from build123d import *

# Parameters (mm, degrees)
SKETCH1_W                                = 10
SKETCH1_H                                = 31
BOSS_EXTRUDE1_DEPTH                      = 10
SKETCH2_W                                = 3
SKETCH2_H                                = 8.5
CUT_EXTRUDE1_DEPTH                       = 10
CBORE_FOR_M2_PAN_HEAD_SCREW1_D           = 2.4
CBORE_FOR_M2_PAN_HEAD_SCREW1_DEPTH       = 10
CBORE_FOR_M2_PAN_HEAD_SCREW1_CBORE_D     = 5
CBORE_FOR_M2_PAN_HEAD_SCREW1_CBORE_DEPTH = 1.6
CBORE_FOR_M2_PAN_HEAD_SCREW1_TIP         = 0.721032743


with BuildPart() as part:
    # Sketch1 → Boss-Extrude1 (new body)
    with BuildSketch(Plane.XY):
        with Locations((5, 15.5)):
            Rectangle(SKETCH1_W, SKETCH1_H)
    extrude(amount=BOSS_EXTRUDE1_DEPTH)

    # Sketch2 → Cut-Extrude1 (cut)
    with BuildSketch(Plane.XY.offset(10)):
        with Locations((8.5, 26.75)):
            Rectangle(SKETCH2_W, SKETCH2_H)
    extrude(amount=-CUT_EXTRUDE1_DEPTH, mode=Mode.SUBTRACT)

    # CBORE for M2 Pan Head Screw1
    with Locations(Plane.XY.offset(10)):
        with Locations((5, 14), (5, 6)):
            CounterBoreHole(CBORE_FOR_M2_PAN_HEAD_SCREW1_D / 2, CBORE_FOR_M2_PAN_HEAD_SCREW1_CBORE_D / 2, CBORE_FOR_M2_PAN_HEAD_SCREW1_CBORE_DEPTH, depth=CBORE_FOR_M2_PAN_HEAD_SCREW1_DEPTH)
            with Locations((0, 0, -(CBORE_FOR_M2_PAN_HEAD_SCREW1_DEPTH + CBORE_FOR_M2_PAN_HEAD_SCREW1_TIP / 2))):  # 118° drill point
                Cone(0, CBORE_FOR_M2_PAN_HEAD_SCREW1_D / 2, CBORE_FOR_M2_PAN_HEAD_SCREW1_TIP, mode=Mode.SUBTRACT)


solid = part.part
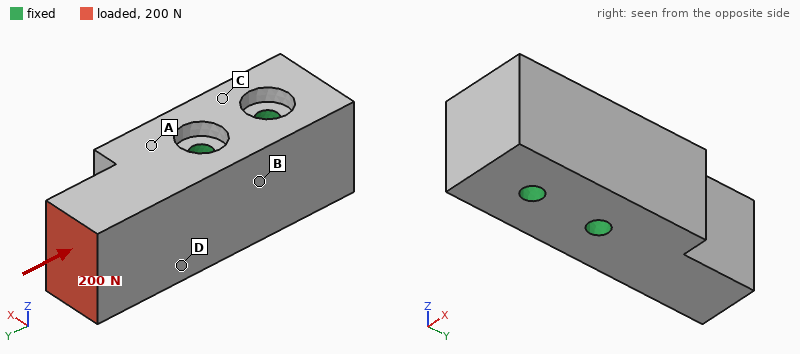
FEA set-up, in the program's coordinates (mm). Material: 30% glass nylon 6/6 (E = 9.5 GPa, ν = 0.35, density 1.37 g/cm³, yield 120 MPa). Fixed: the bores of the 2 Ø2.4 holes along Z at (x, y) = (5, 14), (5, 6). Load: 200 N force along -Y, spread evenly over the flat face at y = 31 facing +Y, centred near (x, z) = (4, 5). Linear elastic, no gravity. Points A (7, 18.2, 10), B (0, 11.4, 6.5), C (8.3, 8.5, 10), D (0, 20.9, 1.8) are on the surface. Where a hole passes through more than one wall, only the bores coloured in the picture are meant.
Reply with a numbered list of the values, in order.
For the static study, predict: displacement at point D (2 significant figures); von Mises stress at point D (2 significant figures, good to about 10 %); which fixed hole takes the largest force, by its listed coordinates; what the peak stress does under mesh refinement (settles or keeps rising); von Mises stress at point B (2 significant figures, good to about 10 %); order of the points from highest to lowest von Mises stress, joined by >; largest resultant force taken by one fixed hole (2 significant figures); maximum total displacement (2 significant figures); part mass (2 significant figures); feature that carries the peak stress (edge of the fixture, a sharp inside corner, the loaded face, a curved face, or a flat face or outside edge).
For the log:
1. 4.4 µm
2. 3.2 MPa
3. (5, 14)
4. keeps rising
5. 2.0 MPa
6. D > B > A > C
7. 160 N
8. 10 µm
9. 3.7 g
10. edge of the fixture
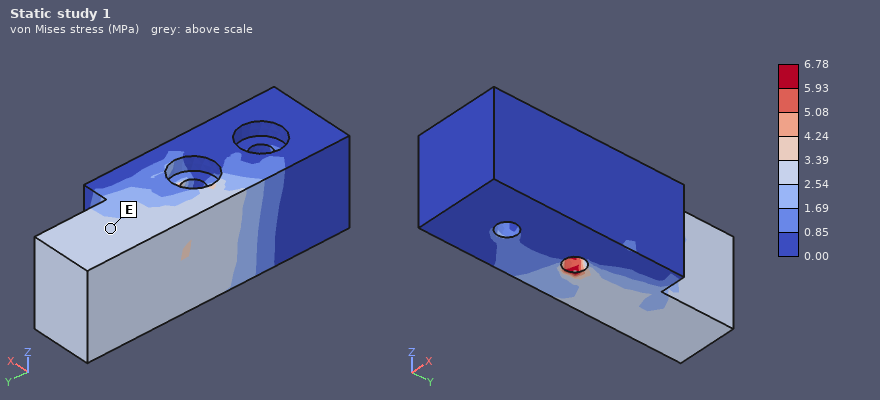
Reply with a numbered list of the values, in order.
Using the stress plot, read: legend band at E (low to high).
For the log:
1. 2.54 to 3.39 MPa
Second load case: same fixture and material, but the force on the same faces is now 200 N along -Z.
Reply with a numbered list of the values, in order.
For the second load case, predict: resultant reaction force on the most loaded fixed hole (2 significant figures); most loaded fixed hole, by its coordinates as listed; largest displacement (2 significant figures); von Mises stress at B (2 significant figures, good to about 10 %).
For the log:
1. 290 N
2. (5, 14)
3. 84 µm
4. 5.4 MPa
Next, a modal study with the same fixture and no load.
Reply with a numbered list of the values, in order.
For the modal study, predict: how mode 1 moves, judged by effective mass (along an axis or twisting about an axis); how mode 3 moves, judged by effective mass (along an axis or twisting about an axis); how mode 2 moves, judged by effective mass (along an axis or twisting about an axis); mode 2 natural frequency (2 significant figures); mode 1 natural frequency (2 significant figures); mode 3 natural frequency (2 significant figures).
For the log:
1. along X
2. twisting about Y
3. along Z
4. 12 kHz
5. 10 kHz
6. 23 kHz
